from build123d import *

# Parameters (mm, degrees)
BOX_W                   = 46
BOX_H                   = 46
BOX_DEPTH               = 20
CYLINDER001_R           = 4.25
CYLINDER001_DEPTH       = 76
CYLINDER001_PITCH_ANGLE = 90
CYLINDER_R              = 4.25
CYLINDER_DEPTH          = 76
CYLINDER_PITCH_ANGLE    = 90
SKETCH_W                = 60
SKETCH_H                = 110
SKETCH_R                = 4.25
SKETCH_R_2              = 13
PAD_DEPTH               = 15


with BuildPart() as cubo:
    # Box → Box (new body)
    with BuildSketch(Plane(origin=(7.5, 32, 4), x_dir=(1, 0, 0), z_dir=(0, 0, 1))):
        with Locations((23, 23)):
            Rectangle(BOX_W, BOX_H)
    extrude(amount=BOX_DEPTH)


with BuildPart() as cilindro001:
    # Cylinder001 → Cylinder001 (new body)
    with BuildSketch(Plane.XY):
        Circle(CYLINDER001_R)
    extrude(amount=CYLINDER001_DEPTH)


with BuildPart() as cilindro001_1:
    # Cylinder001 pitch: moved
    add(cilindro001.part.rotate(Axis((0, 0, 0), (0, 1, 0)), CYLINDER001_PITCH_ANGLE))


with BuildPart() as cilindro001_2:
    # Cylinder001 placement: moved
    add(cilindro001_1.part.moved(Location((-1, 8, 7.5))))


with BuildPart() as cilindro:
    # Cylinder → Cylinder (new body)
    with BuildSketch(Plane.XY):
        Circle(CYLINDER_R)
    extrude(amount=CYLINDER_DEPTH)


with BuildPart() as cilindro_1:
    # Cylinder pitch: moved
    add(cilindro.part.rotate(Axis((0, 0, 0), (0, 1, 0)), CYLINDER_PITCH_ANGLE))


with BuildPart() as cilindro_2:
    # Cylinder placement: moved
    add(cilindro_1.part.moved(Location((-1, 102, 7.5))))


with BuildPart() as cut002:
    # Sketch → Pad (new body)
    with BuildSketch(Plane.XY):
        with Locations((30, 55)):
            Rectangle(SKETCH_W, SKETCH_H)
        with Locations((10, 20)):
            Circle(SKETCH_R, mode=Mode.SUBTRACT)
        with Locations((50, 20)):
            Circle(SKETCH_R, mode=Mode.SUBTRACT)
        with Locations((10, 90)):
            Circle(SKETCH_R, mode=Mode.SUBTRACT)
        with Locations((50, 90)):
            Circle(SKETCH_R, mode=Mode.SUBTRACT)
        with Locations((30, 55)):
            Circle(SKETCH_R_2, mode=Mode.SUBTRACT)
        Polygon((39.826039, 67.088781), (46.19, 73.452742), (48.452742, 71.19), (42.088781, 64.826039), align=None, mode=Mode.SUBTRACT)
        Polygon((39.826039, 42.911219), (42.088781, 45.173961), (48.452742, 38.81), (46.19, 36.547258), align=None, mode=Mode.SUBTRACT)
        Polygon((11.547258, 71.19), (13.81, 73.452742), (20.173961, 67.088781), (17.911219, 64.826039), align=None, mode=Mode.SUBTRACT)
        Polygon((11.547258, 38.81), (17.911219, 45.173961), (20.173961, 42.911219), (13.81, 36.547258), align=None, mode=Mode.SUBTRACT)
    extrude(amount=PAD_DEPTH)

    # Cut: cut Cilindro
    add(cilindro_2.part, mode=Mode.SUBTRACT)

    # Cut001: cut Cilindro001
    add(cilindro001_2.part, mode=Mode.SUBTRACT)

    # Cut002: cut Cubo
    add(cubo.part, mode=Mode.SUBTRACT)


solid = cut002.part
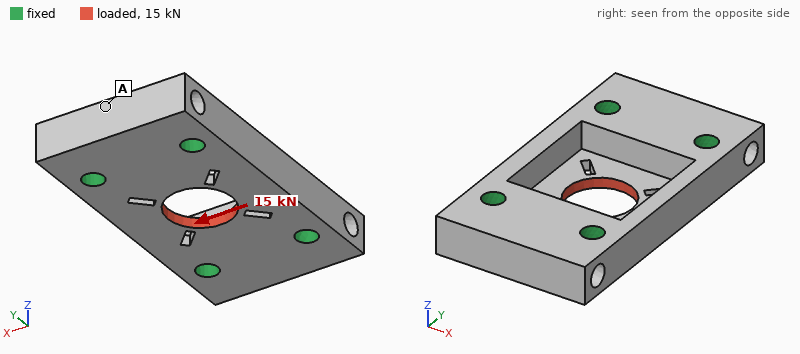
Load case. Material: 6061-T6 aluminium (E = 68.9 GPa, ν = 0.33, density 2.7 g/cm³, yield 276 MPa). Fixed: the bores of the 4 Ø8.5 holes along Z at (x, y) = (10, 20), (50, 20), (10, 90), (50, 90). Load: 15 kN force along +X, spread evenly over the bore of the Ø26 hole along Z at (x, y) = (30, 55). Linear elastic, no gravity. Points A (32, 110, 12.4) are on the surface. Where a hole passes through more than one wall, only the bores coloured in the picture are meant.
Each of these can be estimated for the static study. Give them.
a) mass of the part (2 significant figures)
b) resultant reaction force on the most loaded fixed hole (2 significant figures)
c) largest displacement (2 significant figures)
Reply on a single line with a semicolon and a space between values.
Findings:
170 g; 4.5 kN; 44 µm
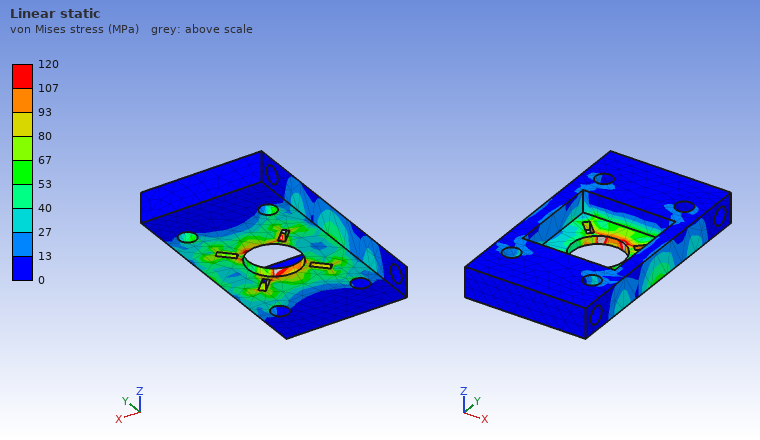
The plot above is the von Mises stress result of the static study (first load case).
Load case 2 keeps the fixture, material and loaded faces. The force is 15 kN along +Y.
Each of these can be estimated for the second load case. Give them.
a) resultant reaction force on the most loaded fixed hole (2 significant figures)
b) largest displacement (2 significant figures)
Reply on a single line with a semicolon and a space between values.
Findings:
3.9 kN; 23 µm
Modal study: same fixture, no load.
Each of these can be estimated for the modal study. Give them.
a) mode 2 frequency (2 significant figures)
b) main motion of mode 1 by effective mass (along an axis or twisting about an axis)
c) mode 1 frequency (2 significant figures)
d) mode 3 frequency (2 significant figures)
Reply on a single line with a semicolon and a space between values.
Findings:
14 kHz; along Z; 13 kHz; 15 kHz
